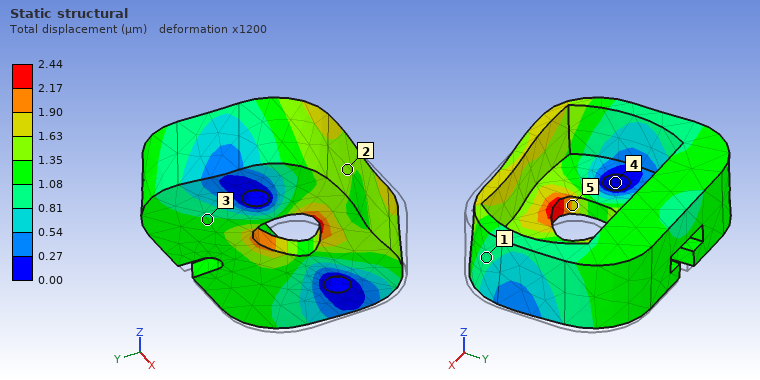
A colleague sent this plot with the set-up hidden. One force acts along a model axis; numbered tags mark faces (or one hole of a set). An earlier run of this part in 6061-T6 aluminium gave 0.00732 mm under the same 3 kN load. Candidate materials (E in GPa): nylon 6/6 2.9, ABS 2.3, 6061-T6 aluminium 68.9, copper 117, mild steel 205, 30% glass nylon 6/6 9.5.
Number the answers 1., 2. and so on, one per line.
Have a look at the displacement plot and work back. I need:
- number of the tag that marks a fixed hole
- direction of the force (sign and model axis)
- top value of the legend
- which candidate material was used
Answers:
1. 4
2. -X
3. 2.44 µm
4. mild steel
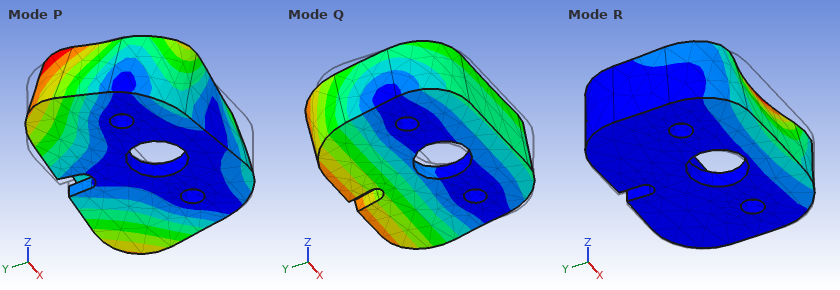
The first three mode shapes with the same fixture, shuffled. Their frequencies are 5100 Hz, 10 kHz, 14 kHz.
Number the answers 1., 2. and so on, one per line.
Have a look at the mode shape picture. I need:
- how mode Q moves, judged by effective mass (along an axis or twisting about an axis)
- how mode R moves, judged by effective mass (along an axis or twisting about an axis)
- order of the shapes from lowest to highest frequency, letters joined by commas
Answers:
1. along Z
2. along Z
3. Q, P, R
